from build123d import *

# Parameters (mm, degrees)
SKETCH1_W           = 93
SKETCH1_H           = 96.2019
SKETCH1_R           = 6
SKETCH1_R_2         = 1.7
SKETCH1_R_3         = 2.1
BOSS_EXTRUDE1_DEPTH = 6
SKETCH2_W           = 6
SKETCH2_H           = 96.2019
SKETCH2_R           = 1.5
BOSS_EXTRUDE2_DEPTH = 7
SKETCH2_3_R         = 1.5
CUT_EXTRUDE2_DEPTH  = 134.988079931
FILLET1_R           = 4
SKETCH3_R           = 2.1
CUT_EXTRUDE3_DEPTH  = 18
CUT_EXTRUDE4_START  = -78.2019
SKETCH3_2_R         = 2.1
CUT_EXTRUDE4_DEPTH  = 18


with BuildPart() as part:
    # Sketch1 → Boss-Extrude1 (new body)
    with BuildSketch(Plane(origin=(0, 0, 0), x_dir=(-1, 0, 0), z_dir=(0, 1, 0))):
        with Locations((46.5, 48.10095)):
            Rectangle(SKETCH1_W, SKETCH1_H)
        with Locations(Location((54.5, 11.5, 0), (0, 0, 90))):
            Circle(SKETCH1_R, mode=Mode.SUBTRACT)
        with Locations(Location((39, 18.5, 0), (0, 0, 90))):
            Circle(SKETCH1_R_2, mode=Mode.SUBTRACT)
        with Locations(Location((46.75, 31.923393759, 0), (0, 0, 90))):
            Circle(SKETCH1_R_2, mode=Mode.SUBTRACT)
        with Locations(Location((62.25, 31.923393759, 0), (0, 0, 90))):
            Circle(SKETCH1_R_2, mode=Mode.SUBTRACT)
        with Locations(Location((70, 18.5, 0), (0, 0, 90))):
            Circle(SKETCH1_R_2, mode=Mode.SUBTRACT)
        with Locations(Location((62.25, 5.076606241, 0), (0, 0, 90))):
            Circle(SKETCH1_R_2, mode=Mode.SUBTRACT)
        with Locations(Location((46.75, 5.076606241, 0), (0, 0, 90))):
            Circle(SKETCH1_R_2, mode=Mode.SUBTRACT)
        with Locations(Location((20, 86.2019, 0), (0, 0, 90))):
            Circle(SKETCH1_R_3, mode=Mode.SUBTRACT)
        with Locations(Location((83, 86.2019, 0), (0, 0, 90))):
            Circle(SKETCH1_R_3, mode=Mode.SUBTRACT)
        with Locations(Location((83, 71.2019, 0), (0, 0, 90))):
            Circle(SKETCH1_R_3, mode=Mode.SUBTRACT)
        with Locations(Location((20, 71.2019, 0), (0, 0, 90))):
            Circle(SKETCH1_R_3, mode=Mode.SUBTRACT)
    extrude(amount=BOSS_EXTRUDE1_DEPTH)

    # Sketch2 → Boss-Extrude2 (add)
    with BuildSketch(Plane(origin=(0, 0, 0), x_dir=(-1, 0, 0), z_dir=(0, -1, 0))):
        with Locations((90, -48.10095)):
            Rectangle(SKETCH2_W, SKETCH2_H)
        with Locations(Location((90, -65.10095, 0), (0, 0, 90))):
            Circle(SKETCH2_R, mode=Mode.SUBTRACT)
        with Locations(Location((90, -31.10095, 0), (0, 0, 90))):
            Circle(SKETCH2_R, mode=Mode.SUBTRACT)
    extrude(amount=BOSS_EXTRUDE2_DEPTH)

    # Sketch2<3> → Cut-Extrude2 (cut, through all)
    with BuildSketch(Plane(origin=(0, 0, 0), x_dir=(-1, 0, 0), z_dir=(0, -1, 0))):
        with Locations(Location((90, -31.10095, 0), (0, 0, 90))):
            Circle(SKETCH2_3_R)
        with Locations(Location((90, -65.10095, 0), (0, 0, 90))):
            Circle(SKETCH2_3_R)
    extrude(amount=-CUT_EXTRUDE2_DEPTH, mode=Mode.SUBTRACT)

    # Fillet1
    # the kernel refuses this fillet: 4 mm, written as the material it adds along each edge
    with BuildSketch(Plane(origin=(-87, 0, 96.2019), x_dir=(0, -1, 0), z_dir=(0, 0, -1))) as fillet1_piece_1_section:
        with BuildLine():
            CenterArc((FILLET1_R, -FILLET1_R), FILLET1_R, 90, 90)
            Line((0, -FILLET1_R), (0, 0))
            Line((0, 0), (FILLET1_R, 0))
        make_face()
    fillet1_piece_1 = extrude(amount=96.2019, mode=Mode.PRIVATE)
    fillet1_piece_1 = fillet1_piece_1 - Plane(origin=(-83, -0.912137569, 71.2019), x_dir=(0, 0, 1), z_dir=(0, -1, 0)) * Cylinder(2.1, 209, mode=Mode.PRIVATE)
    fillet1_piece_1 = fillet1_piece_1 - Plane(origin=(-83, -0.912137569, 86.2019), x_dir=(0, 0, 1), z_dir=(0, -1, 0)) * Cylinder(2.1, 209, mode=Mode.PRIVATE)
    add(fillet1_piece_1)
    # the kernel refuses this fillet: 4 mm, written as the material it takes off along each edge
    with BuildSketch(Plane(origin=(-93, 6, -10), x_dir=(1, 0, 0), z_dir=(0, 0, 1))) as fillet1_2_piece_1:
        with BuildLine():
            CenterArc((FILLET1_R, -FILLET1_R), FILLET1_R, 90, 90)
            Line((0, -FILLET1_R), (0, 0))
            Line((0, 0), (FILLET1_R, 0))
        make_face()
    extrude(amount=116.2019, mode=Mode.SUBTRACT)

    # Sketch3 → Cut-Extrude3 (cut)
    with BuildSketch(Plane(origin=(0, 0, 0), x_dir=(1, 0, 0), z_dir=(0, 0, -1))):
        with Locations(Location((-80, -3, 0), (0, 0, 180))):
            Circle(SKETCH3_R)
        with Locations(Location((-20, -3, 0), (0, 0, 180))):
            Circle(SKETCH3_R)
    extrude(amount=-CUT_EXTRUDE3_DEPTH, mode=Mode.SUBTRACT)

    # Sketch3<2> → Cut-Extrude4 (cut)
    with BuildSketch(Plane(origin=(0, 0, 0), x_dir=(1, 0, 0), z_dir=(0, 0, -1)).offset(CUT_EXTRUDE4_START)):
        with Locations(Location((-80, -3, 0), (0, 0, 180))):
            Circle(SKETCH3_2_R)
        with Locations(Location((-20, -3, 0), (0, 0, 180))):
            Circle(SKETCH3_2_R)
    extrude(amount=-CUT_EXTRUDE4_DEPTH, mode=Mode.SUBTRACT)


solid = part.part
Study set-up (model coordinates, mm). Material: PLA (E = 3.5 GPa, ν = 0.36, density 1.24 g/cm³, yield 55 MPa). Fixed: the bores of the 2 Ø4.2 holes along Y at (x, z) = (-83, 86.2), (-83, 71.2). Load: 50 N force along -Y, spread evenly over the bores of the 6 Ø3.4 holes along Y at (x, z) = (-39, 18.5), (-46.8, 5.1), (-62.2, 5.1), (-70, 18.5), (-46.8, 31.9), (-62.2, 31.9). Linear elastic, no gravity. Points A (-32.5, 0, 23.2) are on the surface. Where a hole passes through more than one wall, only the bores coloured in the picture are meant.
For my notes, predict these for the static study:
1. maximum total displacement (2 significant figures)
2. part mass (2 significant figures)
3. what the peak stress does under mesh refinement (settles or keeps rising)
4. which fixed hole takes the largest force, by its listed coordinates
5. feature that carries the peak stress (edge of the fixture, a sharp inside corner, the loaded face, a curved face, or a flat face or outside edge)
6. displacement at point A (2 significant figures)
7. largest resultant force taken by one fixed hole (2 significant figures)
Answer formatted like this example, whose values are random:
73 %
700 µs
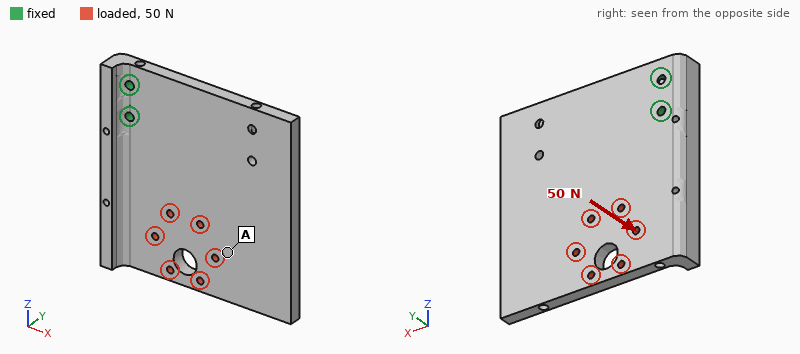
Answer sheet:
1.6 mm
69 g
keeps rising
(-83, 71.2)
edge of the fixture
0.93 mm
150 N
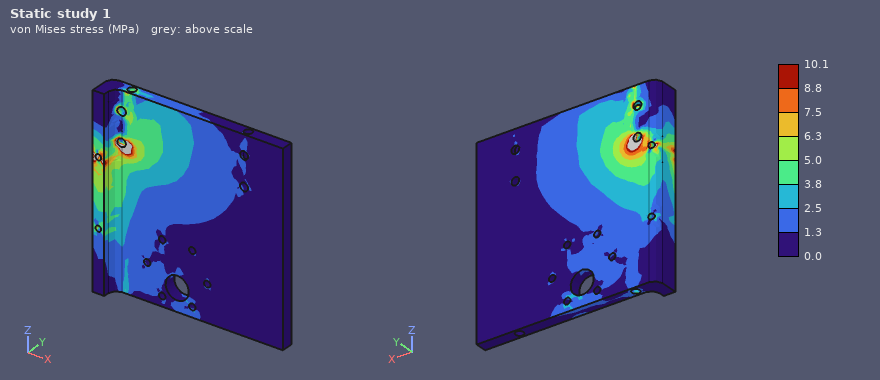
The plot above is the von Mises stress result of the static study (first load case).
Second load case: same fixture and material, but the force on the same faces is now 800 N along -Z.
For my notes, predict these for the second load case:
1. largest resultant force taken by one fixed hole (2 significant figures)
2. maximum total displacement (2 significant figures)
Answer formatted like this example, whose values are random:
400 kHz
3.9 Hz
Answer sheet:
1.4 kN
1.0 mm
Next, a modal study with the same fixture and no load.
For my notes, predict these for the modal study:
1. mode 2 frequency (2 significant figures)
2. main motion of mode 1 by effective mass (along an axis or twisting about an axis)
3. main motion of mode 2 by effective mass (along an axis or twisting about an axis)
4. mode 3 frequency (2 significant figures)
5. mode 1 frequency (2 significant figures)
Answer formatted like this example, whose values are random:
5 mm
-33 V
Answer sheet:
340 Hz
along Y
twisting about X
510 Hz
170 Hz
